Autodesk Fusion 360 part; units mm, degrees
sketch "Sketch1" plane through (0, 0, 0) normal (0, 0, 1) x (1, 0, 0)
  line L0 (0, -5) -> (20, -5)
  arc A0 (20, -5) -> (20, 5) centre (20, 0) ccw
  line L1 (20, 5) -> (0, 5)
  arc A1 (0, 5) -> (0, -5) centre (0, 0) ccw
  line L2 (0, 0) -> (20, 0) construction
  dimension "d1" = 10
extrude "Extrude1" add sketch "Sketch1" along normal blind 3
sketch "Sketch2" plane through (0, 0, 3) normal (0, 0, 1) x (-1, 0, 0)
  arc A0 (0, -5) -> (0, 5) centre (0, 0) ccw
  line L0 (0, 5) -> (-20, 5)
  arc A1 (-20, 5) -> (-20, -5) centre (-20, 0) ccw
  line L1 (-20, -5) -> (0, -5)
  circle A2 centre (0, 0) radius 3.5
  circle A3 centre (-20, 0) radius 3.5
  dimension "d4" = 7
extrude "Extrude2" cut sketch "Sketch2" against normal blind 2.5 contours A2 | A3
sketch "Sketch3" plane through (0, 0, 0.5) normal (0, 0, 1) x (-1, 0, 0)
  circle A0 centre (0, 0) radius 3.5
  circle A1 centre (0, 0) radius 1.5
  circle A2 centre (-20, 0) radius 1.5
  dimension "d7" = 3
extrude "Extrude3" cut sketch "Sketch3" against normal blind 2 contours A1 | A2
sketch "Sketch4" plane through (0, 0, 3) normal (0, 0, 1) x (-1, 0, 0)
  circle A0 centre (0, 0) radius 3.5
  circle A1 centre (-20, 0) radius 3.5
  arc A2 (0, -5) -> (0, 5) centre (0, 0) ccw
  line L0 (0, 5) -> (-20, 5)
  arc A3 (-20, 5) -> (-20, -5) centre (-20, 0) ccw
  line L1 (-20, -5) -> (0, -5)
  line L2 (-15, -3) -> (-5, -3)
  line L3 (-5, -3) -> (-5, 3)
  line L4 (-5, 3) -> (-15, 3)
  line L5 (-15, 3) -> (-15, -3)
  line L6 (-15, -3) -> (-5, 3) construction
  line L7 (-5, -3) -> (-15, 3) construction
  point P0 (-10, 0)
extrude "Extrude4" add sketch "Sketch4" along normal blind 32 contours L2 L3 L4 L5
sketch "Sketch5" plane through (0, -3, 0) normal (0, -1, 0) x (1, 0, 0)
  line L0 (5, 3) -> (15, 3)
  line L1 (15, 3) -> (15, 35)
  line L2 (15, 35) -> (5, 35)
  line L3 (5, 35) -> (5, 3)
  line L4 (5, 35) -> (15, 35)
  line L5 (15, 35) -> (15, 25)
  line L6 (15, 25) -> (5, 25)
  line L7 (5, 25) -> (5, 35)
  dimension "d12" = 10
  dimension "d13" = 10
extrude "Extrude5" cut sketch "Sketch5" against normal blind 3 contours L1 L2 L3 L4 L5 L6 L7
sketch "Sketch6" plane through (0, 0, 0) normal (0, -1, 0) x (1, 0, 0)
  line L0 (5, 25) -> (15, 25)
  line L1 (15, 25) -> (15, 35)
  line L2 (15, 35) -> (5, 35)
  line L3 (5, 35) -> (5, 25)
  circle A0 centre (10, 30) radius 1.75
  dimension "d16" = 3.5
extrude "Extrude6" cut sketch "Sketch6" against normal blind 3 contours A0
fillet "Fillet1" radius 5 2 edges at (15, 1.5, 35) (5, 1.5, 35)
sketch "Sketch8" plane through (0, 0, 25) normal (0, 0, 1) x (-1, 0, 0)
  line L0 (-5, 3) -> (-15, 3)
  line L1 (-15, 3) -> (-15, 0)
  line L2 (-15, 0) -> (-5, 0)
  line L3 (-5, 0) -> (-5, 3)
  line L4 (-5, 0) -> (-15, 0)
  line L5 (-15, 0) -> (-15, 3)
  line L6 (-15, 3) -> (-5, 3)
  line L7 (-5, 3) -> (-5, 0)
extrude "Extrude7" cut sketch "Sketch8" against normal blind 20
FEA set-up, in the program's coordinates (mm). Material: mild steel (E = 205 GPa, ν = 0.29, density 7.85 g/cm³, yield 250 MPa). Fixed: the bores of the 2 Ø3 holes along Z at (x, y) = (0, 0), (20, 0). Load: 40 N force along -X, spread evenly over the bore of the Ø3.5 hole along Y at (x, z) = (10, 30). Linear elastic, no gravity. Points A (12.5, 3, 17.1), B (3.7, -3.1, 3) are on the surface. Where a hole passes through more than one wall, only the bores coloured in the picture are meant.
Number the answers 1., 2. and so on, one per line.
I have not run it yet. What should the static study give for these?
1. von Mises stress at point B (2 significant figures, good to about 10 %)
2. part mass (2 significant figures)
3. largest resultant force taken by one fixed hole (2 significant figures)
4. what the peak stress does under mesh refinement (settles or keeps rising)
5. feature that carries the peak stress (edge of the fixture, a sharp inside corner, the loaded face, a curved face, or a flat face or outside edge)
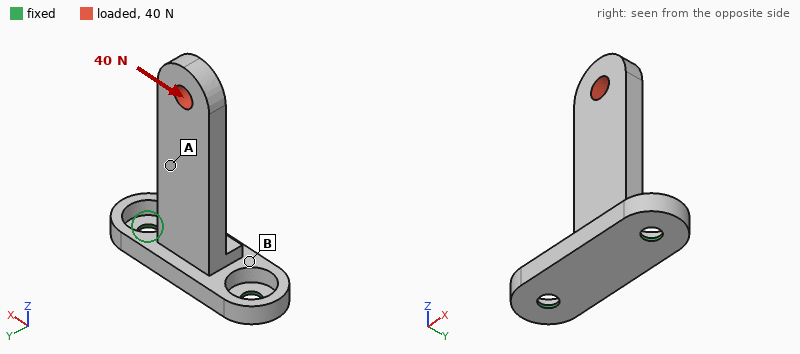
1. 19 MPa
2. 13 g
3. 65 N
4. keeps rising
5. edge of the fixture
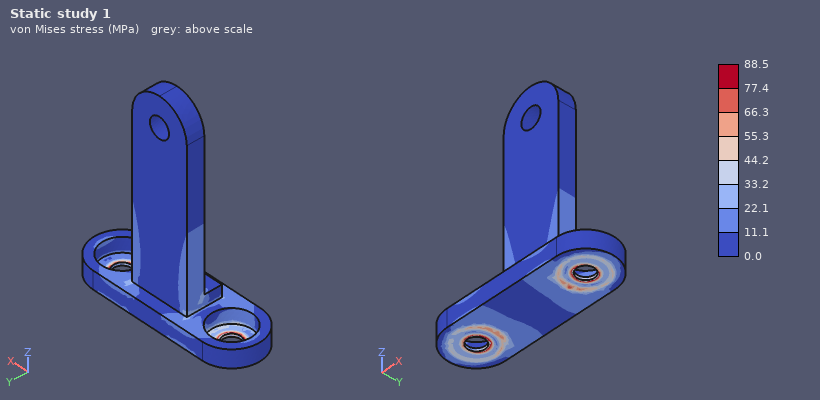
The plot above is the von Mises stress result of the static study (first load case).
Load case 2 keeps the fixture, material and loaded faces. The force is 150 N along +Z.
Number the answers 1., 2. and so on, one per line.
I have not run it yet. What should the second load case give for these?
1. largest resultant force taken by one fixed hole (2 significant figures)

1. 110 N
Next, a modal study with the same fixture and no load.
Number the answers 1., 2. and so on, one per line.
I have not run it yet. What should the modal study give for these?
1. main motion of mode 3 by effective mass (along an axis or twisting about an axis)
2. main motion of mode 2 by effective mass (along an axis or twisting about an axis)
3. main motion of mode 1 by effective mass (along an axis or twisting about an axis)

1. along Z
2. along X
3. along Y
